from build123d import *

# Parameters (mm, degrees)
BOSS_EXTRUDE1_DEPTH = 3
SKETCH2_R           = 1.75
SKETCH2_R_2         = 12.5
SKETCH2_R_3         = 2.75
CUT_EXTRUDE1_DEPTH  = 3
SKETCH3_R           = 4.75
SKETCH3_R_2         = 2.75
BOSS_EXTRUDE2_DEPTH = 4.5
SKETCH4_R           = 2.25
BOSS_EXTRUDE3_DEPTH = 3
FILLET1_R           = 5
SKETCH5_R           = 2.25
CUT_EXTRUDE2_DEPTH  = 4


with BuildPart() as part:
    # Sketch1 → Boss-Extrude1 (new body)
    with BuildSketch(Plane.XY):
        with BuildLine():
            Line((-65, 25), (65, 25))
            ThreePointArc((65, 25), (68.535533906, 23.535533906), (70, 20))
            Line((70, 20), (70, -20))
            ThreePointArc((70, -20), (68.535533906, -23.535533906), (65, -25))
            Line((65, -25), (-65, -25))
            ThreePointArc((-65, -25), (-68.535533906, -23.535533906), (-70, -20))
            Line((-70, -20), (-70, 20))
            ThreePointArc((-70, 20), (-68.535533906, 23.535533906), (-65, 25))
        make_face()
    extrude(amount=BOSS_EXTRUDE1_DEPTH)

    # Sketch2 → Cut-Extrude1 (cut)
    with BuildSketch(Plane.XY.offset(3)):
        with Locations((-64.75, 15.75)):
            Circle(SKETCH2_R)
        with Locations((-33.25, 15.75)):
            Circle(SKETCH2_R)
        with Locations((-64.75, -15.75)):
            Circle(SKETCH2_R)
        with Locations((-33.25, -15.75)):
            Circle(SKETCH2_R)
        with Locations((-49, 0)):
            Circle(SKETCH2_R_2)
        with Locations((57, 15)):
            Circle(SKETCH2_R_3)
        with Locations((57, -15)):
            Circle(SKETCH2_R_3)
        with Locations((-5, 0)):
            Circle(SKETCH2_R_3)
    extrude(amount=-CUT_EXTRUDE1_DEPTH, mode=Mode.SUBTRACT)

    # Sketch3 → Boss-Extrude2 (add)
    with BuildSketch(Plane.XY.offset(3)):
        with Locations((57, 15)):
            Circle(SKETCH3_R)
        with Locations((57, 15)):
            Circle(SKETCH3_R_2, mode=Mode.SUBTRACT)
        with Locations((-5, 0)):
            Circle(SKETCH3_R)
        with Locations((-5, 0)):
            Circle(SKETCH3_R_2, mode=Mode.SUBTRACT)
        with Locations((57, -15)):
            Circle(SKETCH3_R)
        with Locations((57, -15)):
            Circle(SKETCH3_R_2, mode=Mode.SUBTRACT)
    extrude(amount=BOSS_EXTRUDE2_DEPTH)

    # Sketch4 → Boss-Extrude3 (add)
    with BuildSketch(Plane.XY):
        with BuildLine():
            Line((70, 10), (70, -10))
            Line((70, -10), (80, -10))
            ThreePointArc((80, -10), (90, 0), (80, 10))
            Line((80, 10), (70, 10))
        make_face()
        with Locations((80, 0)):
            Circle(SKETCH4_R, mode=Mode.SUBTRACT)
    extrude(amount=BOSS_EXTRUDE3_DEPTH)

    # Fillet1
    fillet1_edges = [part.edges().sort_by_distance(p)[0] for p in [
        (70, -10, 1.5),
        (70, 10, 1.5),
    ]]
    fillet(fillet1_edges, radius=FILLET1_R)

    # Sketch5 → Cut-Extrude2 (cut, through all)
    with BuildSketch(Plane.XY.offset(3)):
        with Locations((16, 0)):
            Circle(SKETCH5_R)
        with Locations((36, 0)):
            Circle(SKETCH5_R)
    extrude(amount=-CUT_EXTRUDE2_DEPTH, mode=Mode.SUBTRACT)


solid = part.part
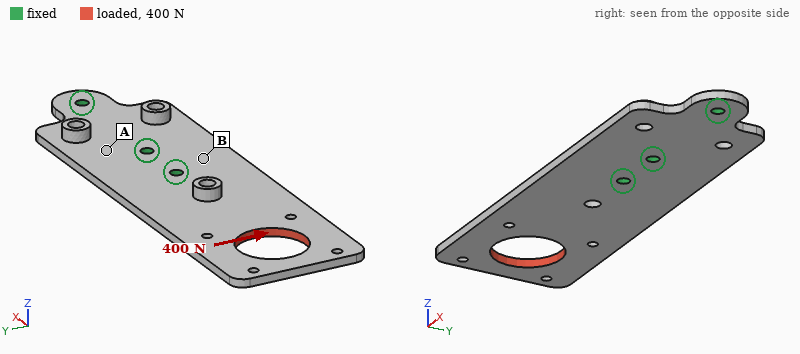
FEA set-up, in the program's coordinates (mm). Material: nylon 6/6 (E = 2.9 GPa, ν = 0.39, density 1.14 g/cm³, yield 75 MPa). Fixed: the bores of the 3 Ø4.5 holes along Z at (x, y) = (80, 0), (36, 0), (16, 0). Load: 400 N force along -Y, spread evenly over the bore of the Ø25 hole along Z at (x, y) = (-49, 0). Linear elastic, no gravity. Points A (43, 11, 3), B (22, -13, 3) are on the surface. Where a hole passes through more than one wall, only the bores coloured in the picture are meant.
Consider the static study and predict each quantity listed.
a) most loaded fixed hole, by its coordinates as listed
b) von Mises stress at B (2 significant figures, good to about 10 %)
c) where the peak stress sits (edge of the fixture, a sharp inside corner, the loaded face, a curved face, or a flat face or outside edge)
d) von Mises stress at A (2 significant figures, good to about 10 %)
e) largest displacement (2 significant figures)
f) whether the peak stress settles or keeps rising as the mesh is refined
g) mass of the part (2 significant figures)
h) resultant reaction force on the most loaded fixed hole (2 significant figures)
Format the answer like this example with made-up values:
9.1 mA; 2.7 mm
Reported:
(16, 0); 13 MPa; edge of the fixture; 5.6 MPa; 1.8 mm; keeps rising; 24 g; 1.0 kN
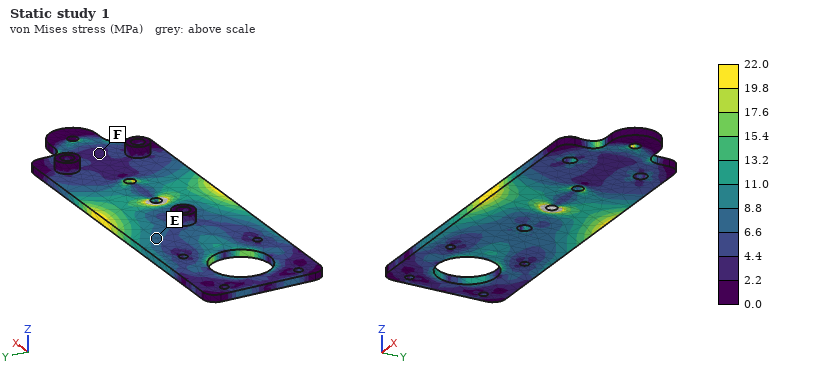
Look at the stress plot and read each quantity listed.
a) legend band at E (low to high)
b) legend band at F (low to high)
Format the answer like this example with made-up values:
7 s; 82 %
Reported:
6.6 to 8.8 MPa; 2.2 to 4.4 MPa
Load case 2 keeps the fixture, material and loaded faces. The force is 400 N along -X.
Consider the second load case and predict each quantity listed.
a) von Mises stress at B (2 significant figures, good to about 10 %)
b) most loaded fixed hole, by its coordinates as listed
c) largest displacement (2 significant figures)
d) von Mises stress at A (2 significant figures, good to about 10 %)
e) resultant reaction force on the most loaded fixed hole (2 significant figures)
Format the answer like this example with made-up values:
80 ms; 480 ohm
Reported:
1.8 MPa; (16, 0); 0.15 mm; 0.90 MPa; 250 N
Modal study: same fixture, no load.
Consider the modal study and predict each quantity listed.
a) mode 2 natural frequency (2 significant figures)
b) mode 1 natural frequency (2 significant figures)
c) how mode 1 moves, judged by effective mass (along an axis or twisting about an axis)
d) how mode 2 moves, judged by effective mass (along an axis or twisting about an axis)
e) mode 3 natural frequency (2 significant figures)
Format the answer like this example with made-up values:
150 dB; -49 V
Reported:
330 Hz; 120 Hz; along Z; twisting about X; 580 Hz
